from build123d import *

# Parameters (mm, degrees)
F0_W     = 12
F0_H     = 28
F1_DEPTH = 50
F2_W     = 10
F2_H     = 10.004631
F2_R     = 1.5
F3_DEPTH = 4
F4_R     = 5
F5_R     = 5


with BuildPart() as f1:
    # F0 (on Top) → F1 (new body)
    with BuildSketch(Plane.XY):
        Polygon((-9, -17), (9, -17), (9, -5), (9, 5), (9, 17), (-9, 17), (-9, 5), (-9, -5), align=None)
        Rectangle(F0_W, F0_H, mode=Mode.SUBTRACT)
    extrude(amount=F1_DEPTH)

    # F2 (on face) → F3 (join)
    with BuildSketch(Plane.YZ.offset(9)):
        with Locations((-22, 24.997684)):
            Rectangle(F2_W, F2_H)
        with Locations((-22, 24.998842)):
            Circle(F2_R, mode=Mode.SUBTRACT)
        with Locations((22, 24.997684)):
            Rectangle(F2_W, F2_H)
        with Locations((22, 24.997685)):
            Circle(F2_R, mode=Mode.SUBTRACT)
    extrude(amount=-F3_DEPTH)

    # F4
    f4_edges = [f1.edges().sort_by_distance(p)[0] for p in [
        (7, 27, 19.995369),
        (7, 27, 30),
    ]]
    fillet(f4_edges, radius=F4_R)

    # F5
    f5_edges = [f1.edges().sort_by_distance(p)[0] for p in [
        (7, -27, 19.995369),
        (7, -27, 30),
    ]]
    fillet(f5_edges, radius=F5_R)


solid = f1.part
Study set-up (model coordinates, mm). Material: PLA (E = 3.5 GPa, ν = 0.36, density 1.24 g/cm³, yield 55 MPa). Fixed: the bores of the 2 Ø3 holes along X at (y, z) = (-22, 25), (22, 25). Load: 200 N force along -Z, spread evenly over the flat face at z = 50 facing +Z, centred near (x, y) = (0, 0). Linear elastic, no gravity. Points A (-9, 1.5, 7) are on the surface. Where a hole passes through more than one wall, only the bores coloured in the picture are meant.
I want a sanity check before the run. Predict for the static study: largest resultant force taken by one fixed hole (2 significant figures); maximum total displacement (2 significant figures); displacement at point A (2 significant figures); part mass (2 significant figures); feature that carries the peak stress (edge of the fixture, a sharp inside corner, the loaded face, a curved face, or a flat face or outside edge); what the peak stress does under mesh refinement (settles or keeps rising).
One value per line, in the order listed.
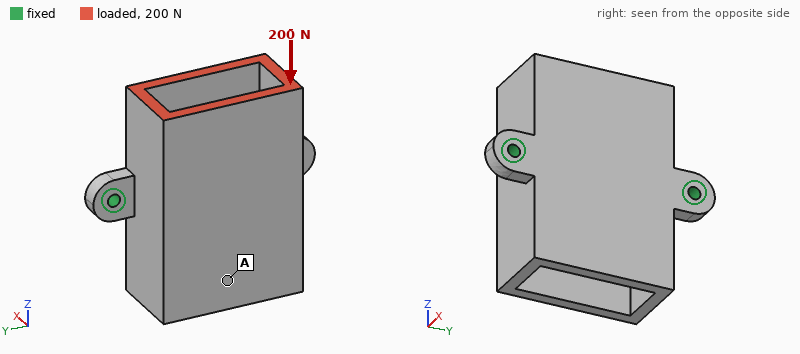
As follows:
100 N
0.51 mm
0.41 mm
18 g
edge of the fixture
keeps rising
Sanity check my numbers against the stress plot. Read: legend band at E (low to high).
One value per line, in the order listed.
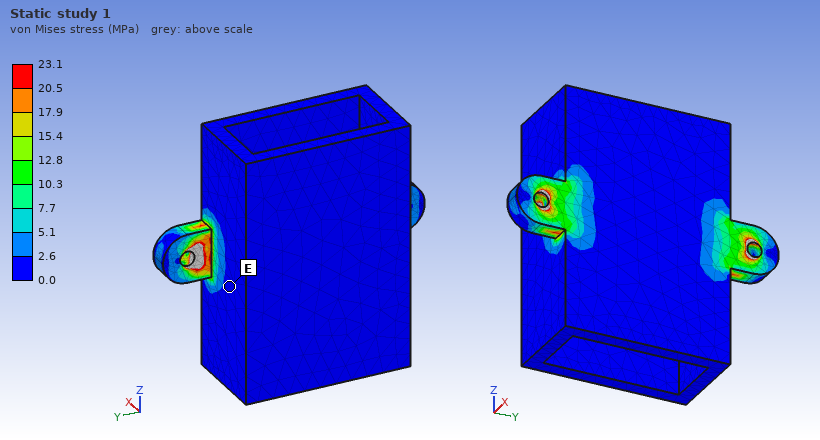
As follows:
0.0 to 2.6 MPa
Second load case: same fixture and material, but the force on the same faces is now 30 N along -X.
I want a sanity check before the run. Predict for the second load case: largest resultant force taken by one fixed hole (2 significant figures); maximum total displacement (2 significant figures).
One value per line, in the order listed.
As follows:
15 N
0.29 mm
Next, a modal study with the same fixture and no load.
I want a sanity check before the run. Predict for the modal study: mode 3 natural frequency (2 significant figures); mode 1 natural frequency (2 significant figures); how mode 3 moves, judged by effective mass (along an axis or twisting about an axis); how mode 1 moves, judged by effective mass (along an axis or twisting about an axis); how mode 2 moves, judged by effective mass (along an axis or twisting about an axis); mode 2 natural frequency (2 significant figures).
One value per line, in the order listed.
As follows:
2400 Hz
640 Hz
twisting about X
along Z
along Y
2100 Hz
